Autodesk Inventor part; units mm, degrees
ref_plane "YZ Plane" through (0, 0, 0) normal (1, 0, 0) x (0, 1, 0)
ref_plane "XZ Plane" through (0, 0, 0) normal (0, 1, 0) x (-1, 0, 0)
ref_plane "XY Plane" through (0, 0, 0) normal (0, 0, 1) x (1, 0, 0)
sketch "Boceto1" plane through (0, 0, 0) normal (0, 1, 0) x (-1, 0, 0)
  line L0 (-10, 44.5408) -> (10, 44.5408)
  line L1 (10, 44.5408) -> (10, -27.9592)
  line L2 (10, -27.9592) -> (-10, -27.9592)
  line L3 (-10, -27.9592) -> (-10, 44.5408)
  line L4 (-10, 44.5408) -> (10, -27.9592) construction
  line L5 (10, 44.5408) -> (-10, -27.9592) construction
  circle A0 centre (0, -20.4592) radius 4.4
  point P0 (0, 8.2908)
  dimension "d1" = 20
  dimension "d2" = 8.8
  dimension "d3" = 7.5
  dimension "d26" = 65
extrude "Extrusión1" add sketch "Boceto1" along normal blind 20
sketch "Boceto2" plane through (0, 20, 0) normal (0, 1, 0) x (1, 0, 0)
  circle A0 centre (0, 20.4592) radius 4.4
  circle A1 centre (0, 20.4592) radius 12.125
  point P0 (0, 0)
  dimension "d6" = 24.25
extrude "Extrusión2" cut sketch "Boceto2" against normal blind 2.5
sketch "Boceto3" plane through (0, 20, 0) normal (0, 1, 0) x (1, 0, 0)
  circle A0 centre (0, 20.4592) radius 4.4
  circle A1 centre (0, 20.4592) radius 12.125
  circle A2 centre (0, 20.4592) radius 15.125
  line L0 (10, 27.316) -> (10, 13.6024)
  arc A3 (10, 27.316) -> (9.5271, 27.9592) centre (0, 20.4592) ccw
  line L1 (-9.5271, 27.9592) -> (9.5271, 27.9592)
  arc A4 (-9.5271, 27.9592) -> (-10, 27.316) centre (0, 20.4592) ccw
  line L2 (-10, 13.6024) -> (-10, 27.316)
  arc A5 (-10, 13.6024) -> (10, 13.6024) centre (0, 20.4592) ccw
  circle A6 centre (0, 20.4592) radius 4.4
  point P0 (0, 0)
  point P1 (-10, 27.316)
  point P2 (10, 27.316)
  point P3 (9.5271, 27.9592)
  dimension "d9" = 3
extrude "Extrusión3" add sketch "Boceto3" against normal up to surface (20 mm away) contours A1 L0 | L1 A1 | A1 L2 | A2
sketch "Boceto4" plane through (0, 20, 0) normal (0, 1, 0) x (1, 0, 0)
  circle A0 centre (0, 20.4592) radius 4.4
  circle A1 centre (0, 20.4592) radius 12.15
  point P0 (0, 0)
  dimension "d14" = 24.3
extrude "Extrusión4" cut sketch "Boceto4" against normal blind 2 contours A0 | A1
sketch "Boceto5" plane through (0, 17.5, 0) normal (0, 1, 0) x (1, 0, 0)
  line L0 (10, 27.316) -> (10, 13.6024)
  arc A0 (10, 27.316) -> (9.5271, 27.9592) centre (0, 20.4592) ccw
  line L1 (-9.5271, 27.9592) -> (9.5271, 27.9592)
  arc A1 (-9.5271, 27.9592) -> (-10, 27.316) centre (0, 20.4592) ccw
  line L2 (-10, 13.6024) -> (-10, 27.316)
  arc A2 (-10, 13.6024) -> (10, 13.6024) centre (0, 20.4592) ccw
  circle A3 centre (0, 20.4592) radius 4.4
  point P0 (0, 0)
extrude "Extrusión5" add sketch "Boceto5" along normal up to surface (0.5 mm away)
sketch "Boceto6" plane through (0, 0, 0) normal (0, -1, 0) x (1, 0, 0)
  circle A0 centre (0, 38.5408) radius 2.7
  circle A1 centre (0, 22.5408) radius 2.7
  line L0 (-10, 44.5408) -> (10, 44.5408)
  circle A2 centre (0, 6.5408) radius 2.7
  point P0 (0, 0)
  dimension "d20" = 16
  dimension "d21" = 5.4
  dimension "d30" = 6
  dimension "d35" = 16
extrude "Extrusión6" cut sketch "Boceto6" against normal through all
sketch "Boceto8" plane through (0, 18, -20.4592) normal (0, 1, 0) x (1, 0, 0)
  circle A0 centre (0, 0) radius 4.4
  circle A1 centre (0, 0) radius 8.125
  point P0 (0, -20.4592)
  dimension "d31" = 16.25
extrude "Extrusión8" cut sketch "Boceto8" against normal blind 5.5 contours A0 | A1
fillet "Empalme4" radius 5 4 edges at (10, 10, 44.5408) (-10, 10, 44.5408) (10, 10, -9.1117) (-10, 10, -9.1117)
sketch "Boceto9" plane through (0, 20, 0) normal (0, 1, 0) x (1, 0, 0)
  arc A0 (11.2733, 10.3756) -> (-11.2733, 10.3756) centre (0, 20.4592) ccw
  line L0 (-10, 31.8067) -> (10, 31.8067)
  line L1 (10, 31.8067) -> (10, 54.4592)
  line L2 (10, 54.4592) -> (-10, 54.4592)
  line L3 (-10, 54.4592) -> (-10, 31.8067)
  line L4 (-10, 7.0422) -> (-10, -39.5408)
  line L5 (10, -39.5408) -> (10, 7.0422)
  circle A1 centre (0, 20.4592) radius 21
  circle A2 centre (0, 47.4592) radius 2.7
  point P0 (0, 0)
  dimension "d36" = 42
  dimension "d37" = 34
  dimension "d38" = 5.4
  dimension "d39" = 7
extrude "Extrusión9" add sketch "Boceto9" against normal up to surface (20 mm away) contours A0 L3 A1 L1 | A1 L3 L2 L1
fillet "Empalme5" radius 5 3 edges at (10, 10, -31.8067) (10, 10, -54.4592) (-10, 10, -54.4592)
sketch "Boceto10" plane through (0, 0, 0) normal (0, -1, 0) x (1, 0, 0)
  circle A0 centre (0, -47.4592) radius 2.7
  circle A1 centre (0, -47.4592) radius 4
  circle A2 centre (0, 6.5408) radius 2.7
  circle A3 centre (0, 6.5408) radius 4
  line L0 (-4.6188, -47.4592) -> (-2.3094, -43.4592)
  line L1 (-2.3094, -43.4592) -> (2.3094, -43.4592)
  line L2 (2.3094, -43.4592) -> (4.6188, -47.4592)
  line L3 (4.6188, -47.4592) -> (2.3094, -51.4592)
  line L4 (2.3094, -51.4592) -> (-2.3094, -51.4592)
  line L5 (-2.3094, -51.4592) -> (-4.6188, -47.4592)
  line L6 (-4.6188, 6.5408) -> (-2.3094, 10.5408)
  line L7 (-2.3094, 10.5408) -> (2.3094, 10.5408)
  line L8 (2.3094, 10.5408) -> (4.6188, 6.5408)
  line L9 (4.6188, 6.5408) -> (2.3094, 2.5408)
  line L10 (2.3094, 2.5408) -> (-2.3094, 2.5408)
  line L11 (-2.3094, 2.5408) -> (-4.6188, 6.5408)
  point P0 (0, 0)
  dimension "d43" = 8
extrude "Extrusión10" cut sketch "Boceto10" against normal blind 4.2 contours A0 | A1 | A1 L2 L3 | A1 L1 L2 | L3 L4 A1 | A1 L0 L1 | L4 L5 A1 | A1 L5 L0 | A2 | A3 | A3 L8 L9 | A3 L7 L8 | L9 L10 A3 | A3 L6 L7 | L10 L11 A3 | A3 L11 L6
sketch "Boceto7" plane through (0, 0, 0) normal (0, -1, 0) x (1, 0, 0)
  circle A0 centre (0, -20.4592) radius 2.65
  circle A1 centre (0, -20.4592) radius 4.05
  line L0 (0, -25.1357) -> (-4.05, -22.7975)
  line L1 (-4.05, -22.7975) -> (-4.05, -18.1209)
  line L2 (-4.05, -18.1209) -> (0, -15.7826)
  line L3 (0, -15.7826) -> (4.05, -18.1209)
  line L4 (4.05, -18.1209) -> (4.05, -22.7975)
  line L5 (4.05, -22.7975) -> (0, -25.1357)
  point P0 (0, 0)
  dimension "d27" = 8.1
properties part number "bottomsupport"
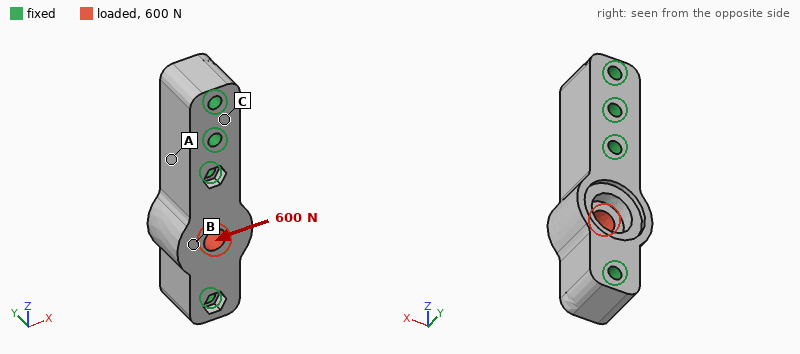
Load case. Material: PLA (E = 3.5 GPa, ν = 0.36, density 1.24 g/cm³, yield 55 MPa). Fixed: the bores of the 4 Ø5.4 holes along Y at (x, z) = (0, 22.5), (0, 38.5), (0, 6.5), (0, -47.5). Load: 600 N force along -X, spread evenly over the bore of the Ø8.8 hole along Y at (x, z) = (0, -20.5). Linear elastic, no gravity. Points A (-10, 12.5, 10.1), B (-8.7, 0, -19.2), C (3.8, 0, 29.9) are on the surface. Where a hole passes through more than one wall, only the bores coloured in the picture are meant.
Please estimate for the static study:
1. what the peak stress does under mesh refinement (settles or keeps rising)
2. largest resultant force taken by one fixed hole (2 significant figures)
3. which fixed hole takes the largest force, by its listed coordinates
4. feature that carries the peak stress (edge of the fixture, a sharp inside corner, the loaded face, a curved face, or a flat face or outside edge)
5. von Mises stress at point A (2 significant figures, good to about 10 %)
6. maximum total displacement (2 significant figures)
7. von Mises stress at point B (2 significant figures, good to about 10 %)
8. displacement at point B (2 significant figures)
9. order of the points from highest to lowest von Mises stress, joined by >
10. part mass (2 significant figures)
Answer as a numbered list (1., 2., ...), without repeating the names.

1. keeps rising
2. 390 N
3. (0, 6.5)
4. edge of the fixture
5. 1.4 MPa
6. 42 µm
7. 2.1 MPa
8. 40 µm
9. B > A > C
10. 46 g
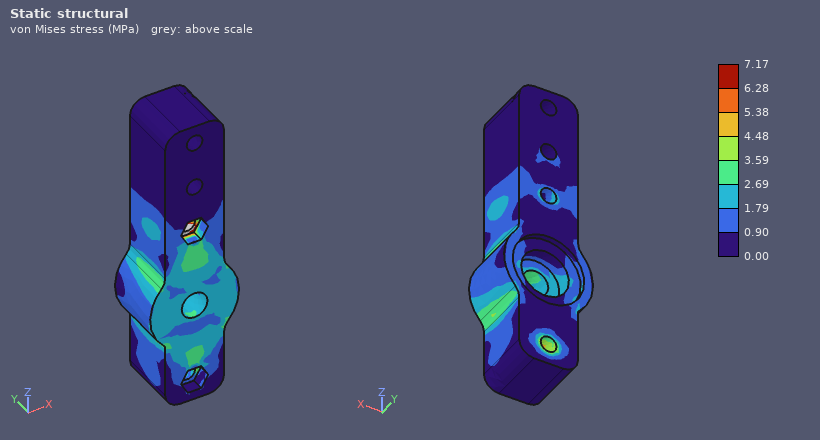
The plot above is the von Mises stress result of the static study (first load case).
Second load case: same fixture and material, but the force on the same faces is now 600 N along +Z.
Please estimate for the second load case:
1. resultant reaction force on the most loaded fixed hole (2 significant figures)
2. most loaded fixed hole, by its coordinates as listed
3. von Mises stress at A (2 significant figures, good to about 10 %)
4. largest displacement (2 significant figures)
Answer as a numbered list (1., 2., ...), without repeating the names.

1. 290 N
2. (0, -47.5)
3. 0.40 MPa
4. 9.8 µm
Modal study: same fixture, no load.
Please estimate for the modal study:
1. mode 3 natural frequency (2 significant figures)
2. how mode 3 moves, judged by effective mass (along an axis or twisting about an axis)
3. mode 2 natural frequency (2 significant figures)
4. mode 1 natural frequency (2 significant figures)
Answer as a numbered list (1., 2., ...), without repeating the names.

1. 7000 Hz
2. along X
3. 5800 Hz
4. 5800 Hz
